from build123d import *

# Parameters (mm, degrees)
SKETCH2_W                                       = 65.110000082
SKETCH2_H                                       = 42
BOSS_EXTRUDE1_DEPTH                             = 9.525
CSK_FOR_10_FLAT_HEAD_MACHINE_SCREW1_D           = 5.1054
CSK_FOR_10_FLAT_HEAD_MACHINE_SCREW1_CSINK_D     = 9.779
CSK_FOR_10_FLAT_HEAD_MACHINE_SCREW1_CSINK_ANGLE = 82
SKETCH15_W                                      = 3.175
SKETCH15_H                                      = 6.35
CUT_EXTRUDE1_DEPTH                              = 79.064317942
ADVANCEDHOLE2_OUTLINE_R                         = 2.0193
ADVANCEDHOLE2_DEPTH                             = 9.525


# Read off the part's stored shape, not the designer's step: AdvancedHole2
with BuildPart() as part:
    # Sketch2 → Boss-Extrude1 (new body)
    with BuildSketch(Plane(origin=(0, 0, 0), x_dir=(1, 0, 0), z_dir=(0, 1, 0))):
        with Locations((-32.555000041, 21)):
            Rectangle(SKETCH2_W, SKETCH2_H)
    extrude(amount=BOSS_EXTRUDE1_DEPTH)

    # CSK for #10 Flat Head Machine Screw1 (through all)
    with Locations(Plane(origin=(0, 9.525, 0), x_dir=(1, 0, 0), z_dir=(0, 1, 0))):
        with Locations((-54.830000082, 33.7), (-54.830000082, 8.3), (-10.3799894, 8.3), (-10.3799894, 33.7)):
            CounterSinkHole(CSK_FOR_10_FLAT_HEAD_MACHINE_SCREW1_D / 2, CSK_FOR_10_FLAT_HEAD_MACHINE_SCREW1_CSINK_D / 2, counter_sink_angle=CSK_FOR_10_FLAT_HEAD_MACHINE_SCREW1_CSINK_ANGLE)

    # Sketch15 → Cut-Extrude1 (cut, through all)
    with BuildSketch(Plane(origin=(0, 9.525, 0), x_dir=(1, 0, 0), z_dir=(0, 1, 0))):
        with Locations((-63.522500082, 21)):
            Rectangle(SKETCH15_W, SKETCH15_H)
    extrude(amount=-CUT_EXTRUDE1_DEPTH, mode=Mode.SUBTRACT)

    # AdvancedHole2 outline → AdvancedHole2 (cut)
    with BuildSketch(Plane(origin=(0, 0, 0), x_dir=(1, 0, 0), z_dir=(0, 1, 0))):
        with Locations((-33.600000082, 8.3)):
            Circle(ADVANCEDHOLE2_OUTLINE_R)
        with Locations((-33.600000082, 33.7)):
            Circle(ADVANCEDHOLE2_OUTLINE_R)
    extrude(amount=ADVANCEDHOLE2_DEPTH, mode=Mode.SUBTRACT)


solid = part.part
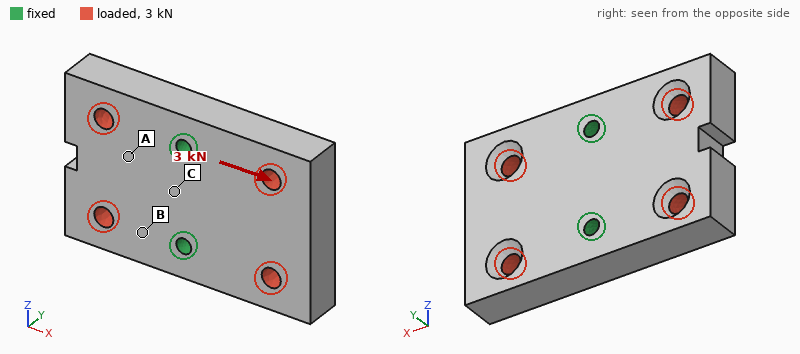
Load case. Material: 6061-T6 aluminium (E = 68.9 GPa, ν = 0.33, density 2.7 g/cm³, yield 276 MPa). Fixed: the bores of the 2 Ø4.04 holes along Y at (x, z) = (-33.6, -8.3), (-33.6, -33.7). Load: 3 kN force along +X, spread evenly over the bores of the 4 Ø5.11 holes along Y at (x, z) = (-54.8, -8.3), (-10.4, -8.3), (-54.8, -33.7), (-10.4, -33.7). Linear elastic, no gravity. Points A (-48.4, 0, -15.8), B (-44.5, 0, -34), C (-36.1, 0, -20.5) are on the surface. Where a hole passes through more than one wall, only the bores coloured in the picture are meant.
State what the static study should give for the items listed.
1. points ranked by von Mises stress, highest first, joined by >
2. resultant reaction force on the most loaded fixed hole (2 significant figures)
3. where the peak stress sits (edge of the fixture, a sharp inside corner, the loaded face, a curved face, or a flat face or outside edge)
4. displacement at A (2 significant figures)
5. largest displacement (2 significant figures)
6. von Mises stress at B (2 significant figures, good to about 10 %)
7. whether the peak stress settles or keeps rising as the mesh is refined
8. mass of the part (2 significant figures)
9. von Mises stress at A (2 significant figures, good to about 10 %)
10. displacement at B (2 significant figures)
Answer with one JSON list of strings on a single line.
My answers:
["B > A > C", "1.5 kN", "edge of the fixture", "2.8 µm", "7.2 µm", "9.2 MPa", "keeps rising", "66 g", "5.0 MPa", "2.1 µm"]
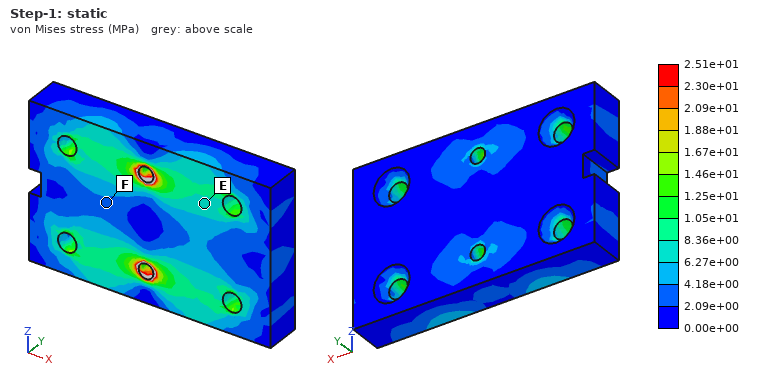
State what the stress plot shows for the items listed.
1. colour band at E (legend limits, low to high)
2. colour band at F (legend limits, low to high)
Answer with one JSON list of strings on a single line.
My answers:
["6.27e+00 to 8.36e+00 MPa", "2.09e+00 to 4.18e+00 MPa"]
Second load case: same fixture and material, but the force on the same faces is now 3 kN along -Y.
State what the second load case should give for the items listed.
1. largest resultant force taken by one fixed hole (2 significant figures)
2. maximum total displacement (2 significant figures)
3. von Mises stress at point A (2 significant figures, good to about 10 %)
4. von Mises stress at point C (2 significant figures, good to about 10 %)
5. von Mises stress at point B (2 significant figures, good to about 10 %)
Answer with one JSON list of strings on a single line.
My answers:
["1.5 kN", "51 µm", "15 MPa", "37 MPa", "23 MPa"]
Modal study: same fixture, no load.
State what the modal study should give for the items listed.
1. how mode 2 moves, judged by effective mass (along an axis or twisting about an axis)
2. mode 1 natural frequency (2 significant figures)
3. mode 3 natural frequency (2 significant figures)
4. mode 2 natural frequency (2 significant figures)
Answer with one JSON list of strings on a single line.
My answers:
["along Y", "5800 Hz", "12 kHz", "7600 Hz"]
